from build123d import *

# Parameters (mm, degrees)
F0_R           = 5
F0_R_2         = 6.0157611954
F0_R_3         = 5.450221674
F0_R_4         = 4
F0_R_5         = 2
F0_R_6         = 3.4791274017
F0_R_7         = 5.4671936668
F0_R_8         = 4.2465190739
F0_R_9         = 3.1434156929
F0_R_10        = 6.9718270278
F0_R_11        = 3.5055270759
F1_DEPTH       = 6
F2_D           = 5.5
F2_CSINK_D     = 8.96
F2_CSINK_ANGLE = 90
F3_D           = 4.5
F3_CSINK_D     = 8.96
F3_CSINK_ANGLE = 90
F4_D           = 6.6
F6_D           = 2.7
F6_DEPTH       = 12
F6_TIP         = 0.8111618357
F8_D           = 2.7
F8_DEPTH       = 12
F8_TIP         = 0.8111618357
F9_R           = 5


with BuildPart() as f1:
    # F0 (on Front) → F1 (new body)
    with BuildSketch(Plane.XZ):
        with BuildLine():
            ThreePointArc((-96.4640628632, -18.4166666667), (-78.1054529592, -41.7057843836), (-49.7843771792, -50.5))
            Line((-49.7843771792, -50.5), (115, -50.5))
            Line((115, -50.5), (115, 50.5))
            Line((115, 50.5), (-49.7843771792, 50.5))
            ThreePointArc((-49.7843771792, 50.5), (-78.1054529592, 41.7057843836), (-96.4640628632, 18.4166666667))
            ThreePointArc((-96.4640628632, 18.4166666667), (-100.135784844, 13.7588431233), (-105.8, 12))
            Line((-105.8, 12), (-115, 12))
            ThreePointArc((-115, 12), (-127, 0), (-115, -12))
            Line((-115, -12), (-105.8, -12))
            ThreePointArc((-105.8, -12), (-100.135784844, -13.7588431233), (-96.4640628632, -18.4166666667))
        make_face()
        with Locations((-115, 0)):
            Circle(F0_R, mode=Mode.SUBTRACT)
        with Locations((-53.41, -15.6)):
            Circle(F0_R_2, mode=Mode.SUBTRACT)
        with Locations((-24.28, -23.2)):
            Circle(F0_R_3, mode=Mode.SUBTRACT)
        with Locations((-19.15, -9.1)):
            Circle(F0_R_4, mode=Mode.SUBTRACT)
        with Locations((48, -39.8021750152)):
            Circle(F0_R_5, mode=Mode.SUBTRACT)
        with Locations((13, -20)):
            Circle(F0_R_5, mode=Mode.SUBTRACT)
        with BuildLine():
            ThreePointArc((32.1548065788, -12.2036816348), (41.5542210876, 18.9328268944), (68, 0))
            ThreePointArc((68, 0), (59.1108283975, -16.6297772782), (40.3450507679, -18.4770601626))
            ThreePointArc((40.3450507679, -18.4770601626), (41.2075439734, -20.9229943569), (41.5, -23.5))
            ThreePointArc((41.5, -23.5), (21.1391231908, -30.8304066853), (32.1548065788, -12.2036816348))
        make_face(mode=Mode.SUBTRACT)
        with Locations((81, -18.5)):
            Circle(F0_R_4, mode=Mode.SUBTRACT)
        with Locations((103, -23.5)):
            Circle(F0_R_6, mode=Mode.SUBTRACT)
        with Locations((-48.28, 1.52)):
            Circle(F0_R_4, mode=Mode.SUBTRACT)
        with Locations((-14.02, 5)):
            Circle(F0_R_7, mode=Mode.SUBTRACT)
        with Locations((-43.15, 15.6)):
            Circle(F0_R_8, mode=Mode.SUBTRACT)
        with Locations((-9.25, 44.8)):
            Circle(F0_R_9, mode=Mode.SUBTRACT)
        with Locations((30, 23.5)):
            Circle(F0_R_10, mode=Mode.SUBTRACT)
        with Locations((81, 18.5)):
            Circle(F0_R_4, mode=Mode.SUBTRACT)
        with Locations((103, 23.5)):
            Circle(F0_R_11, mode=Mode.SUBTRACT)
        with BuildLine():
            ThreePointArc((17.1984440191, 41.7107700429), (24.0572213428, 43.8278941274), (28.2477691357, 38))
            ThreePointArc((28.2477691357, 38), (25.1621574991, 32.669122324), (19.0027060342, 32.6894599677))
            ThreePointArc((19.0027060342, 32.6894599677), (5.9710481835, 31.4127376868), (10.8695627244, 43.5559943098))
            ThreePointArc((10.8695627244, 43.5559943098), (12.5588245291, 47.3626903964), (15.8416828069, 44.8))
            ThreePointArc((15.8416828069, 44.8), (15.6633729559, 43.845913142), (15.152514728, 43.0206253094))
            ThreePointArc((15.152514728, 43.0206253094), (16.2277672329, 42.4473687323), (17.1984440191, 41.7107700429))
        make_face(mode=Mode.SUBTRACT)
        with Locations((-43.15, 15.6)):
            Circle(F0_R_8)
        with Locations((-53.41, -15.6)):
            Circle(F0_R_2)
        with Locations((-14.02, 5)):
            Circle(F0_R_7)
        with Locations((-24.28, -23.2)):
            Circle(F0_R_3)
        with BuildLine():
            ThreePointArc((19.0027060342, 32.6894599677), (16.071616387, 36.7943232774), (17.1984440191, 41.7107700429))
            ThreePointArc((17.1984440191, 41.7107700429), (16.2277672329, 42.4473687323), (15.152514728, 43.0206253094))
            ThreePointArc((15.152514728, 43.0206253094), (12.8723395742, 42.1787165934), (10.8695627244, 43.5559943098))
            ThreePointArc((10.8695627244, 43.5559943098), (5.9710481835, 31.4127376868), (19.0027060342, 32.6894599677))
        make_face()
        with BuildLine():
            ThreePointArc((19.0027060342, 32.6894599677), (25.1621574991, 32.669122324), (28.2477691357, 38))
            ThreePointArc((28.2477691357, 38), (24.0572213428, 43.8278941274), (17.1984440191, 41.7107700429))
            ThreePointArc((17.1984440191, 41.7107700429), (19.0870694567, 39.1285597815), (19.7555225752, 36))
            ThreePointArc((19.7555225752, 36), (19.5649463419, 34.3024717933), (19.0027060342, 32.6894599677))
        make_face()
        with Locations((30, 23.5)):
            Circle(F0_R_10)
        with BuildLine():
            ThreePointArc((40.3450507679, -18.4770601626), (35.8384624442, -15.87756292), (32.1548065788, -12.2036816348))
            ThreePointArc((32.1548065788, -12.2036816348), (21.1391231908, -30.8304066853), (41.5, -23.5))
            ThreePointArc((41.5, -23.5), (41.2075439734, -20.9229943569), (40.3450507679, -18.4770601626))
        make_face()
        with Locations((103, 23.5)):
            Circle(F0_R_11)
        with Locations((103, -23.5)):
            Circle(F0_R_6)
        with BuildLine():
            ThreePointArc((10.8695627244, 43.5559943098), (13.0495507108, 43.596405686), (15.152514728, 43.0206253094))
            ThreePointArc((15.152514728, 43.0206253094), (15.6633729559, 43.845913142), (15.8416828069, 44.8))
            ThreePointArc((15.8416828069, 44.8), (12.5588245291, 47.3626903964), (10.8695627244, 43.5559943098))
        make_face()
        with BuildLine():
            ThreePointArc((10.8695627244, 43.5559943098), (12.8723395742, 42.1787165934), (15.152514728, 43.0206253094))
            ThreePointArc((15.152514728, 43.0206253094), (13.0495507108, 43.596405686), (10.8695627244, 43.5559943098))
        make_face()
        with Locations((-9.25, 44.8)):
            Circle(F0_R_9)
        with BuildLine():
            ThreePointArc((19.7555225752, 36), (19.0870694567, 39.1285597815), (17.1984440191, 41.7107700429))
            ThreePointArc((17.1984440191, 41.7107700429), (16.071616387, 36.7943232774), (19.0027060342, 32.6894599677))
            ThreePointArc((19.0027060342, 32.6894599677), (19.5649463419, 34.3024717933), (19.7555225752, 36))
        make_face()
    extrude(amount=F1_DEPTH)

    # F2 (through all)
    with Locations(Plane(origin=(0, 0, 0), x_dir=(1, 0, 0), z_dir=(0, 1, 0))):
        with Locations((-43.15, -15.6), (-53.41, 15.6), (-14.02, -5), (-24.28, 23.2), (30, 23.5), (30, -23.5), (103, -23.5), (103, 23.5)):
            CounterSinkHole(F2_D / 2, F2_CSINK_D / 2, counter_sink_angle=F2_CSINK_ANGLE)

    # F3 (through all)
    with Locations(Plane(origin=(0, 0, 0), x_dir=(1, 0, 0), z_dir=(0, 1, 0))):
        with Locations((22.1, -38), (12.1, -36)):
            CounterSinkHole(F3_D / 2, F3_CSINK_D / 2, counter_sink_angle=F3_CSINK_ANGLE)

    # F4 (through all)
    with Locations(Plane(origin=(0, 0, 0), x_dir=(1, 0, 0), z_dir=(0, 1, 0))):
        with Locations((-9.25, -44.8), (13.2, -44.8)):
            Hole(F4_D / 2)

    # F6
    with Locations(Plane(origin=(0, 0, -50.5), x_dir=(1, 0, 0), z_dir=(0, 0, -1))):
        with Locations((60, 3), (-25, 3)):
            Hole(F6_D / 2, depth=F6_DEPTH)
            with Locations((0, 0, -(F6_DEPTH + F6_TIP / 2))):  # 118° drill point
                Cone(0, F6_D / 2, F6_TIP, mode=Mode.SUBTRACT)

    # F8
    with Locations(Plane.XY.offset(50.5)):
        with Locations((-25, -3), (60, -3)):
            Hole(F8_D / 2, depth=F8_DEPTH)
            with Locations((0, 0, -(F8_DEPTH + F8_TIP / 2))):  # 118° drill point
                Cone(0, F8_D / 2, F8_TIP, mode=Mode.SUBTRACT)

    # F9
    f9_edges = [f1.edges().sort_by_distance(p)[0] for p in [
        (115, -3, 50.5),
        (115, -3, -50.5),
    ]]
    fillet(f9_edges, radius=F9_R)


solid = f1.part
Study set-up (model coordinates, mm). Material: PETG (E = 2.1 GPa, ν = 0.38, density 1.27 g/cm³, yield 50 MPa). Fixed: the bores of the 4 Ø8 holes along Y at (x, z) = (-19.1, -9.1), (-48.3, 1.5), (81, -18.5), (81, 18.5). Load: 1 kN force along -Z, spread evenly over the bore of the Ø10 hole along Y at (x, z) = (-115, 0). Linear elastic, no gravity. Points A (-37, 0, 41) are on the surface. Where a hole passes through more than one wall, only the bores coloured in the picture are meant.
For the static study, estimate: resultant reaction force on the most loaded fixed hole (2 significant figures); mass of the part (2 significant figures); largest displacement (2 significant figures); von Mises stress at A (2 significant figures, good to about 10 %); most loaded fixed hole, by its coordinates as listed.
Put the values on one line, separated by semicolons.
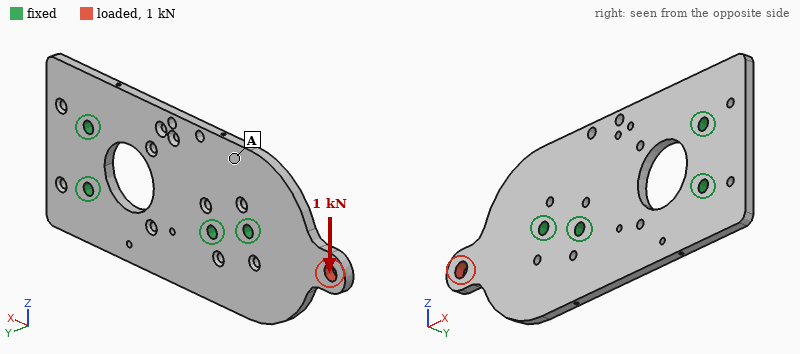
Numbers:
1.6 kN; 150 g; 1.4 mm; 4.4 MPa; (-48.3, 1.5)
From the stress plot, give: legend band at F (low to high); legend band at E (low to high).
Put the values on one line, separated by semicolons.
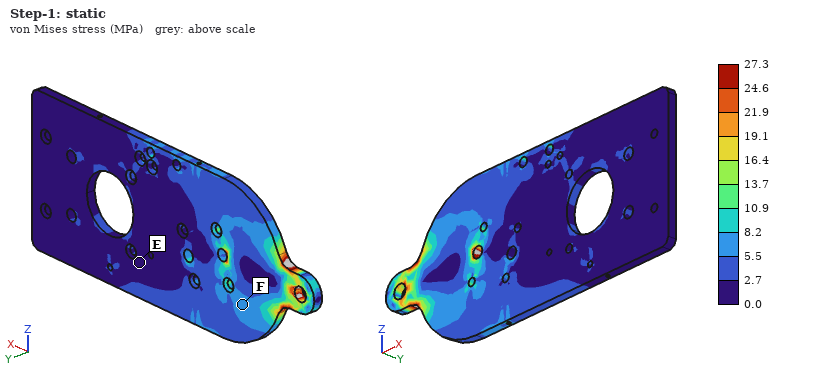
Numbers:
5.5 to 8.2 MPa; 0.0 to 2.7 MPa
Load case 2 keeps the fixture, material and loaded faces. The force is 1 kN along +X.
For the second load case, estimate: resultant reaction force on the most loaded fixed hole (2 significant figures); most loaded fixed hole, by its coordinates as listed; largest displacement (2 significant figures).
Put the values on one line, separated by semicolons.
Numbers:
660 N; (-48.3, 1.5); 0.21 mm
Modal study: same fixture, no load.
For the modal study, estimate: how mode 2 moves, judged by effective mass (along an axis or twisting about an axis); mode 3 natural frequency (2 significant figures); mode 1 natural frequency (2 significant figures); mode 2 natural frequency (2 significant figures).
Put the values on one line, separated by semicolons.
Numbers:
along Y; 540 Hz; 340 Hz; 430 Hz
